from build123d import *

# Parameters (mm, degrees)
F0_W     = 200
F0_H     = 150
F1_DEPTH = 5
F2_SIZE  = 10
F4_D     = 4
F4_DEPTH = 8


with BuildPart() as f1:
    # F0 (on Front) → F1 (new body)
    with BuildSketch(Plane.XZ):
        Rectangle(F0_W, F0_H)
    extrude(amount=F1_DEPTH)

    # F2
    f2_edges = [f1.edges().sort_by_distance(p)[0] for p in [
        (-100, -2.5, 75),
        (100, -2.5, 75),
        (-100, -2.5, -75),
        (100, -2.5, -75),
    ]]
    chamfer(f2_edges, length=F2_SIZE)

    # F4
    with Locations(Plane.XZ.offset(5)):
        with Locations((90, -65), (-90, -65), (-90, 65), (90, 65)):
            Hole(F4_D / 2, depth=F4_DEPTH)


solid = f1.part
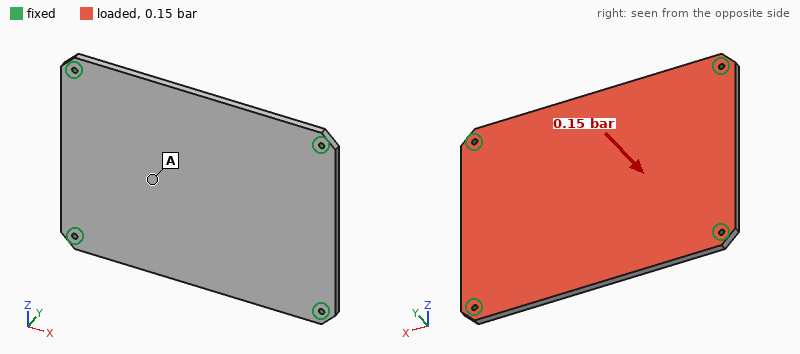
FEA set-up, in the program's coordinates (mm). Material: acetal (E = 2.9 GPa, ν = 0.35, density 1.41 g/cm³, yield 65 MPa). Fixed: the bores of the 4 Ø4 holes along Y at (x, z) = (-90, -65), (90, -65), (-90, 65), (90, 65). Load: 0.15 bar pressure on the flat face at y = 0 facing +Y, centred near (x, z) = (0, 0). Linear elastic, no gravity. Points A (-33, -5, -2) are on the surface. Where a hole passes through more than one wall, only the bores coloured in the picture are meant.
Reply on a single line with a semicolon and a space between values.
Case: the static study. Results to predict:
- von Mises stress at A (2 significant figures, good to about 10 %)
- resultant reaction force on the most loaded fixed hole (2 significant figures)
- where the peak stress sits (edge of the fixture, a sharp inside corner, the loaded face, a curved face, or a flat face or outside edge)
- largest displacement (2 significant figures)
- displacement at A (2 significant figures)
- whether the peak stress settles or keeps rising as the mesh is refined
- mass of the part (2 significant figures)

4.7 MPa; 110 N; edge of the fixture; 2.6 mm; 2.3 mm; keeps rising; 210 g
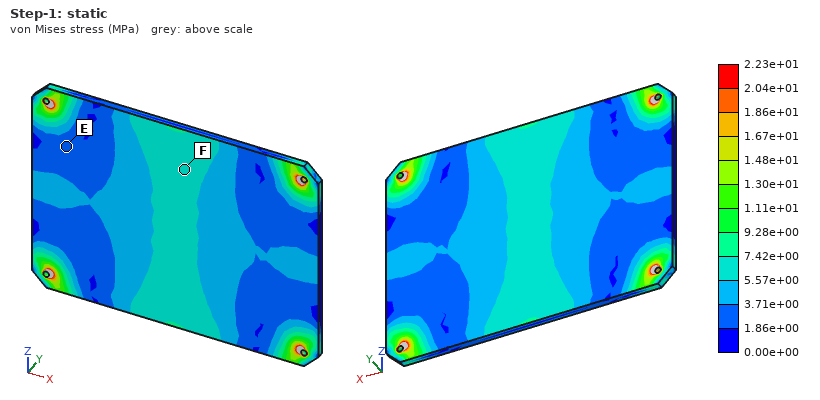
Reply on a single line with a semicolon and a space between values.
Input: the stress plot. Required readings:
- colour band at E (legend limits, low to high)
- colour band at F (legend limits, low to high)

1.86e+00 to 3.71e+00 MPa; 5.57e+00 to 7.42e+00 MPa
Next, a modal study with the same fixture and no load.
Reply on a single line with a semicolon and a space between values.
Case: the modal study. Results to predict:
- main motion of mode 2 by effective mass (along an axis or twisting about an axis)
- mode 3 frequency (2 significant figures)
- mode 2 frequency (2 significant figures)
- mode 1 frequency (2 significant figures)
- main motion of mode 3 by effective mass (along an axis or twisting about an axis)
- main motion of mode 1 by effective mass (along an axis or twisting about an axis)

twisting about X; 380 Hz; 270 Hz; 170 Hz; twisting about Z; along Y
